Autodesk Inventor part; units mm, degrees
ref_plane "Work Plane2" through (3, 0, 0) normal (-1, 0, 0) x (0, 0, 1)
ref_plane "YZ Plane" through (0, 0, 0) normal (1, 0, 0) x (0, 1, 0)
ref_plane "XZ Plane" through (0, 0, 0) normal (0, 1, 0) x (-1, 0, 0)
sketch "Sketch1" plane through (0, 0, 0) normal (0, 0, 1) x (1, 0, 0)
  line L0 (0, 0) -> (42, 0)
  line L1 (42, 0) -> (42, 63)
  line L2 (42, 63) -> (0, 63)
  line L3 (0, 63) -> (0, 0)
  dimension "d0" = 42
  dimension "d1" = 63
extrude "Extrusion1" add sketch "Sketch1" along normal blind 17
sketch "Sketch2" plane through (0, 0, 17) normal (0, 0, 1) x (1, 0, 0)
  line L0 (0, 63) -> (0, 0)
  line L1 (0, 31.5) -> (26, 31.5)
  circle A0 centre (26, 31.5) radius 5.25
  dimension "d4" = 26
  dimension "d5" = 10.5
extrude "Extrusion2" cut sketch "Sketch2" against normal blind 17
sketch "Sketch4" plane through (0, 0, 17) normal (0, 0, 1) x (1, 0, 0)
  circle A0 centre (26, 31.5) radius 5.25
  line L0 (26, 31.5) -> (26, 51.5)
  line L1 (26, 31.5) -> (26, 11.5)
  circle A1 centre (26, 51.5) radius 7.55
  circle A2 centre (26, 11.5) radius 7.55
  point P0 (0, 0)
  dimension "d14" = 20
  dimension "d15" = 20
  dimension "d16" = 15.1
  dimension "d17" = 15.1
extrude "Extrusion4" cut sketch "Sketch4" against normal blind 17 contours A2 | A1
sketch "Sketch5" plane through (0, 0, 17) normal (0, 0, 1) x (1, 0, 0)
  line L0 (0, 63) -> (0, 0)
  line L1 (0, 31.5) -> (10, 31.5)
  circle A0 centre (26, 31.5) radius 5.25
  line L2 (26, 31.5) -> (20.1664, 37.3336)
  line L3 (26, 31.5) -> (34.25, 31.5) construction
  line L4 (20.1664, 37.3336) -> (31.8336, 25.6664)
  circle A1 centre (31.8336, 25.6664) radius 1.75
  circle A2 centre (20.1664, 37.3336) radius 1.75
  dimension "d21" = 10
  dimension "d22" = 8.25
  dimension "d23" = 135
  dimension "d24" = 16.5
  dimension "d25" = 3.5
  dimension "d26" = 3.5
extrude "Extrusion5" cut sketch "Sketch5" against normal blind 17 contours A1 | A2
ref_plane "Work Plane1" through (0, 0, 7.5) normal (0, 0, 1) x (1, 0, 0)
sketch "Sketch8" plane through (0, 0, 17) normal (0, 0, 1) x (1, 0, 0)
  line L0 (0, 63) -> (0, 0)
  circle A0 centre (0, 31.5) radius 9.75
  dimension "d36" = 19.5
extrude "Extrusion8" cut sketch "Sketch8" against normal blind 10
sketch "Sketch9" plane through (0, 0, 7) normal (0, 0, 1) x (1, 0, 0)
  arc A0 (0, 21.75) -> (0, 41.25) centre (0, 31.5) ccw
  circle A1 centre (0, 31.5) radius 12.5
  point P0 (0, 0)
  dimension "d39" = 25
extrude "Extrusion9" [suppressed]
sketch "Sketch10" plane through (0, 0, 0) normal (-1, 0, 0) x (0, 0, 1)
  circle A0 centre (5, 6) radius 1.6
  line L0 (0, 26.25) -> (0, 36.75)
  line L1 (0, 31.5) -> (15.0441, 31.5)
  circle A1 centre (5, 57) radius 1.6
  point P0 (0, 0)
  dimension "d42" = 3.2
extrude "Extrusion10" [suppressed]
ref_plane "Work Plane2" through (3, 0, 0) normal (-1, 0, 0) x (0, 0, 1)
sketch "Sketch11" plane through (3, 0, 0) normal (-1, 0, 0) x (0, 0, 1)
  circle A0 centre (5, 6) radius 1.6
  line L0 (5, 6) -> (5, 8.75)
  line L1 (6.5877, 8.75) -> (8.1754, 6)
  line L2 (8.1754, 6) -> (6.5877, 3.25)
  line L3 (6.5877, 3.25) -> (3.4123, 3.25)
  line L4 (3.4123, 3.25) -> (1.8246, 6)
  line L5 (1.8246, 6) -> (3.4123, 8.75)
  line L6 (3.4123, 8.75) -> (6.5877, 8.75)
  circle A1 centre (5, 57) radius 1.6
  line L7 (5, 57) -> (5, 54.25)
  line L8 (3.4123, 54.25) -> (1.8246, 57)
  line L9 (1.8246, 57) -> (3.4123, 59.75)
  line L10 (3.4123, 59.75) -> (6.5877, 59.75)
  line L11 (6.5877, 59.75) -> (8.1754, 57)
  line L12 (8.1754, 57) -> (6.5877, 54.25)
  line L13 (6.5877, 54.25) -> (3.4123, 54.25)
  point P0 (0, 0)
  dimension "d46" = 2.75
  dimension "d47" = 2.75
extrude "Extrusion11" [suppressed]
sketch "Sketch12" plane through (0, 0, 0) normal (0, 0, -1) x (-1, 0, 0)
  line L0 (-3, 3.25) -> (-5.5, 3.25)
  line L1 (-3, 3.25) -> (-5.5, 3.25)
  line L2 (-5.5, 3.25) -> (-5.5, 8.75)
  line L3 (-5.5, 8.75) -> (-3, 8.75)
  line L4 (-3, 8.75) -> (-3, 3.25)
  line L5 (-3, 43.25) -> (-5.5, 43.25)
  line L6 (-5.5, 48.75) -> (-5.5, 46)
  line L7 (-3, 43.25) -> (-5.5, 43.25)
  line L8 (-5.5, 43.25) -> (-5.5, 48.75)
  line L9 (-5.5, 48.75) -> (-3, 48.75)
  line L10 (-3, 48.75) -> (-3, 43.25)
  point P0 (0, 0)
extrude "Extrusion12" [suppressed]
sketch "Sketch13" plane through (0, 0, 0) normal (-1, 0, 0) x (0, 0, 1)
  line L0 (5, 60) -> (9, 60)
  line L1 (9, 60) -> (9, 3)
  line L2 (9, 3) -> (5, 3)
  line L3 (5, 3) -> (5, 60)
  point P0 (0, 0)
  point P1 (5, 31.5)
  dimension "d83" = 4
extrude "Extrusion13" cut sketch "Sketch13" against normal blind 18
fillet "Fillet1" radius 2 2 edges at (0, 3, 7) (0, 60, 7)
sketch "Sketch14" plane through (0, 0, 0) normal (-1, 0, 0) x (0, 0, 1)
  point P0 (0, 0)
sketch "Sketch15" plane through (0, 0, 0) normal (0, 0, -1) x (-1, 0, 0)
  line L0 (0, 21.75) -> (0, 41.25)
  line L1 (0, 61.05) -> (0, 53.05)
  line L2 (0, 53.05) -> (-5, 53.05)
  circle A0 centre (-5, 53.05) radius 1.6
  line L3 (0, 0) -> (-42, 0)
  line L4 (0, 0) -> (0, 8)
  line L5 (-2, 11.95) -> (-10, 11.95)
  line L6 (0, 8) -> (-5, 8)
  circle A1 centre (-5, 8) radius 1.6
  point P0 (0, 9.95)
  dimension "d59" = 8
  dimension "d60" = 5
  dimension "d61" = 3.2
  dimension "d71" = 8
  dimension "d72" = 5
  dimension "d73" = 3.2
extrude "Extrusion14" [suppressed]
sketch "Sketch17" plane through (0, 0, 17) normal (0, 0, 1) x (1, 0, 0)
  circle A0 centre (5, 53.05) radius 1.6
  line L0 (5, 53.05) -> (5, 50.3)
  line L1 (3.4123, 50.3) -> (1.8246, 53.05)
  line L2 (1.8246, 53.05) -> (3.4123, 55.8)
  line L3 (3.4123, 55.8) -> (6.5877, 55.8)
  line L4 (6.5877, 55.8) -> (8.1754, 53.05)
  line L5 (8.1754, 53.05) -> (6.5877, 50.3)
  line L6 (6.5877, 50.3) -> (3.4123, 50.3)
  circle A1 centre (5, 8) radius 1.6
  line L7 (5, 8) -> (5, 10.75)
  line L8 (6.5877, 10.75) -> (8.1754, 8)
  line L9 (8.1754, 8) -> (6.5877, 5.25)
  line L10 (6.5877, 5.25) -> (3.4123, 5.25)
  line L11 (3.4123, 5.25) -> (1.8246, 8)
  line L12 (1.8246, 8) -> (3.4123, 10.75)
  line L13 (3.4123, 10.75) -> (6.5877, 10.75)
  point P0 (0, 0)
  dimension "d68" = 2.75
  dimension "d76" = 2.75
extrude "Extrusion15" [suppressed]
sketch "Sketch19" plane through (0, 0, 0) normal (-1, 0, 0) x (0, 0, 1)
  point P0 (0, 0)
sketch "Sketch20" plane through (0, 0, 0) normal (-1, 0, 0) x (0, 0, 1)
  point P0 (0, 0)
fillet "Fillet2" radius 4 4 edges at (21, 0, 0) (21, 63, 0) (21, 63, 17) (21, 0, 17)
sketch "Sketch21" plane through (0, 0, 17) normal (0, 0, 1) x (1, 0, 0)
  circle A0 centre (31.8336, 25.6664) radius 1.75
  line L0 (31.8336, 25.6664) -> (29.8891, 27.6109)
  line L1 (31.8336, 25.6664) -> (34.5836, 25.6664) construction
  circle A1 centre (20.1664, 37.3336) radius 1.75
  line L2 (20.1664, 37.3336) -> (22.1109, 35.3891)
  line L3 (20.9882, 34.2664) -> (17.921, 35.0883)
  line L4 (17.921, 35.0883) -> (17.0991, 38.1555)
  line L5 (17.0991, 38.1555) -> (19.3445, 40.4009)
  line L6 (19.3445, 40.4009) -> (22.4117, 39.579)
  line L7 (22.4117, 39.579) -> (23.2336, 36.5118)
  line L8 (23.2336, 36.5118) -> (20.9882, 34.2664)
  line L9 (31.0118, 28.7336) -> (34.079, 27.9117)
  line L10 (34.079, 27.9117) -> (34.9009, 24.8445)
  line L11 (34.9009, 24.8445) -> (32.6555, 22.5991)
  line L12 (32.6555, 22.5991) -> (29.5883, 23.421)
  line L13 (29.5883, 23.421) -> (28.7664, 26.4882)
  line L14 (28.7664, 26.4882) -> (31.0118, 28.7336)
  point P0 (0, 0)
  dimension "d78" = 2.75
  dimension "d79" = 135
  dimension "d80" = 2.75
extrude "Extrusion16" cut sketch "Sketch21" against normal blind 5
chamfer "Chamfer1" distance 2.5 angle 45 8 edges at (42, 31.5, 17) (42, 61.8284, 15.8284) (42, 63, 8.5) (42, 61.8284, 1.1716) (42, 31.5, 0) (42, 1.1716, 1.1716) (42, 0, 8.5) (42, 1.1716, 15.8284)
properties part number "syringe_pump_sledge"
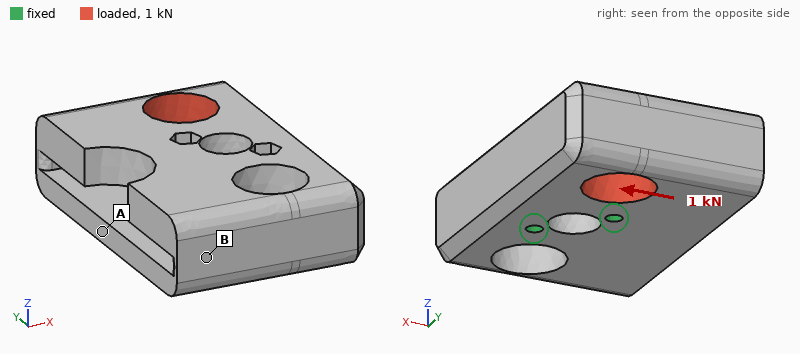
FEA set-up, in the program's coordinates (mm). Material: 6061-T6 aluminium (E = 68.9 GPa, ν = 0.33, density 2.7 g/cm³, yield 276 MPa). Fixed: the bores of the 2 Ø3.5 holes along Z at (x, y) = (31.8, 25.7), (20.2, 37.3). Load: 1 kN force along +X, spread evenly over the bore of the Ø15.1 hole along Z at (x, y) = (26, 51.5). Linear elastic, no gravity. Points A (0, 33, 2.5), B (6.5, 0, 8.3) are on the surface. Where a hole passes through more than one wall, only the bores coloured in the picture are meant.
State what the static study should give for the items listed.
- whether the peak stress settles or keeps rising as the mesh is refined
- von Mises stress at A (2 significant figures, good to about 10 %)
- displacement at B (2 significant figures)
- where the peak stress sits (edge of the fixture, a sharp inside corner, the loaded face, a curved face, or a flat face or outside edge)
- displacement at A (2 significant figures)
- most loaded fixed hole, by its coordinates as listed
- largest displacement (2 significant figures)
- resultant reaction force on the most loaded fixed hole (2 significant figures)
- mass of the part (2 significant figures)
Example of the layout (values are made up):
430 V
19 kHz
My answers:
keeps rising
4.8 MPa
3.7 µm
edge of the fixture
3.6 µm
(20.2, 37.3)
10 µm
1.5 kN
83 g
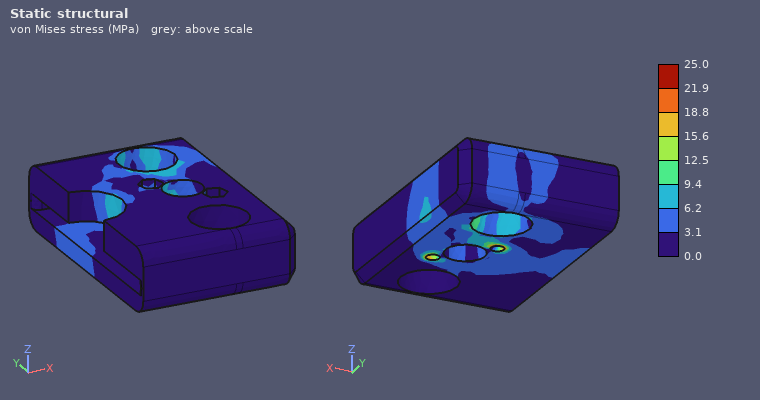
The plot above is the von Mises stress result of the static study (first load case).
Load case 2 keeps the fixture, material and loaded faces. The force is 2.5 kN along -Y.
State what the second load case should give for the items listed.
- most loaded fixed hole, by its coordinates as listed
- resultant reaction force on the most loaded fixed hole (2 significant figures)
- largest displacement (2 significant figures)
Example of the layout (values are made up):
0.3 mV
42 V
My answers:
(20.2, 37.3)
1.4 kN
7.2 µm
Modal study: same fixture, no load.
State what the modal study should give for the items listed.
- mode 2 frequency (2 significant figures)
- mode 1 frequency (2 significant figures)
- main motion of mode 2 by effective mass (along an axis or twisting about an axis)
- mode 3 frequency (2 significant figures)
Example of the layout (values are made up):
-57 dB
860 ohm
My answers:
7800 Hz
5900 Hz
along Z
8500 Hz
